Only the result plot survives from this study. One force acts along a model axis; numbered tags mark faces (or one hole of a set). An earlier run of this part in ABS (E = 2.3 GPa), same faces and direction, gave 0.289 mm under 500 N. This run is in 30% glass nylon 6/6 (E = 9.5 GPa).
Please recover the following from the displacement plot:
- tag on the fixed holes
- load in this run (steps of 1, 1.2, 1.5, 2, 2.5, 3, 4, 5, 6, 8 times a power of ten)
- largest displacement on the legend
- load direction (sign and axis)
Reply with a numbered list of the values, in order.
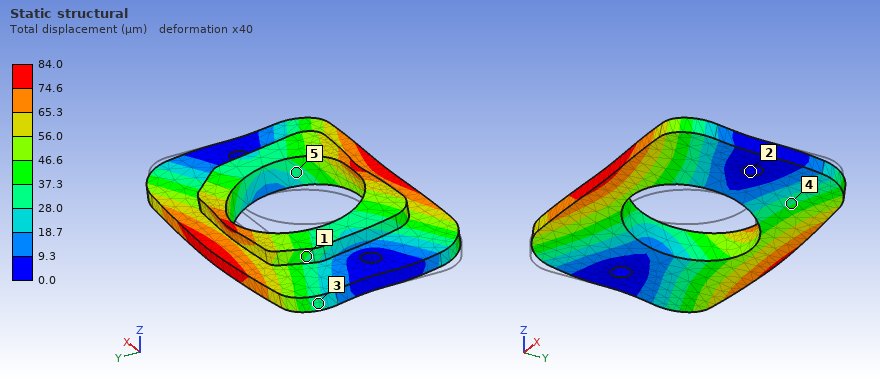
1. 2
2. 600 N
3. 84.0 µm
4. +Y
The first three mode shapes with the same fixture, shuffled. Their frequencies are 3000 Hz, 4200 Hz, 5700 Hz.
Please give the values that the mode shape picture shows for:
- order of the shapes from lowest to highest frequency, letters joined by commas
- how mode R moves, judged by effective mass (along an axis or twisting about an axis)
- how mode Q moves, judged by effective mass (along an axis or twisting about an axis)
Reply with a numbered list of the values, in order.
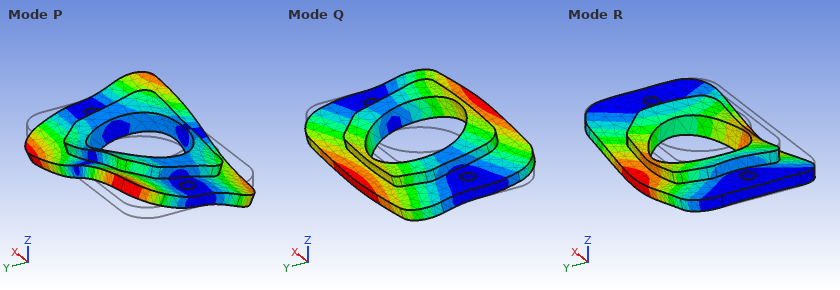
1. Q, R, P
2. along Z
3. twisting about X
